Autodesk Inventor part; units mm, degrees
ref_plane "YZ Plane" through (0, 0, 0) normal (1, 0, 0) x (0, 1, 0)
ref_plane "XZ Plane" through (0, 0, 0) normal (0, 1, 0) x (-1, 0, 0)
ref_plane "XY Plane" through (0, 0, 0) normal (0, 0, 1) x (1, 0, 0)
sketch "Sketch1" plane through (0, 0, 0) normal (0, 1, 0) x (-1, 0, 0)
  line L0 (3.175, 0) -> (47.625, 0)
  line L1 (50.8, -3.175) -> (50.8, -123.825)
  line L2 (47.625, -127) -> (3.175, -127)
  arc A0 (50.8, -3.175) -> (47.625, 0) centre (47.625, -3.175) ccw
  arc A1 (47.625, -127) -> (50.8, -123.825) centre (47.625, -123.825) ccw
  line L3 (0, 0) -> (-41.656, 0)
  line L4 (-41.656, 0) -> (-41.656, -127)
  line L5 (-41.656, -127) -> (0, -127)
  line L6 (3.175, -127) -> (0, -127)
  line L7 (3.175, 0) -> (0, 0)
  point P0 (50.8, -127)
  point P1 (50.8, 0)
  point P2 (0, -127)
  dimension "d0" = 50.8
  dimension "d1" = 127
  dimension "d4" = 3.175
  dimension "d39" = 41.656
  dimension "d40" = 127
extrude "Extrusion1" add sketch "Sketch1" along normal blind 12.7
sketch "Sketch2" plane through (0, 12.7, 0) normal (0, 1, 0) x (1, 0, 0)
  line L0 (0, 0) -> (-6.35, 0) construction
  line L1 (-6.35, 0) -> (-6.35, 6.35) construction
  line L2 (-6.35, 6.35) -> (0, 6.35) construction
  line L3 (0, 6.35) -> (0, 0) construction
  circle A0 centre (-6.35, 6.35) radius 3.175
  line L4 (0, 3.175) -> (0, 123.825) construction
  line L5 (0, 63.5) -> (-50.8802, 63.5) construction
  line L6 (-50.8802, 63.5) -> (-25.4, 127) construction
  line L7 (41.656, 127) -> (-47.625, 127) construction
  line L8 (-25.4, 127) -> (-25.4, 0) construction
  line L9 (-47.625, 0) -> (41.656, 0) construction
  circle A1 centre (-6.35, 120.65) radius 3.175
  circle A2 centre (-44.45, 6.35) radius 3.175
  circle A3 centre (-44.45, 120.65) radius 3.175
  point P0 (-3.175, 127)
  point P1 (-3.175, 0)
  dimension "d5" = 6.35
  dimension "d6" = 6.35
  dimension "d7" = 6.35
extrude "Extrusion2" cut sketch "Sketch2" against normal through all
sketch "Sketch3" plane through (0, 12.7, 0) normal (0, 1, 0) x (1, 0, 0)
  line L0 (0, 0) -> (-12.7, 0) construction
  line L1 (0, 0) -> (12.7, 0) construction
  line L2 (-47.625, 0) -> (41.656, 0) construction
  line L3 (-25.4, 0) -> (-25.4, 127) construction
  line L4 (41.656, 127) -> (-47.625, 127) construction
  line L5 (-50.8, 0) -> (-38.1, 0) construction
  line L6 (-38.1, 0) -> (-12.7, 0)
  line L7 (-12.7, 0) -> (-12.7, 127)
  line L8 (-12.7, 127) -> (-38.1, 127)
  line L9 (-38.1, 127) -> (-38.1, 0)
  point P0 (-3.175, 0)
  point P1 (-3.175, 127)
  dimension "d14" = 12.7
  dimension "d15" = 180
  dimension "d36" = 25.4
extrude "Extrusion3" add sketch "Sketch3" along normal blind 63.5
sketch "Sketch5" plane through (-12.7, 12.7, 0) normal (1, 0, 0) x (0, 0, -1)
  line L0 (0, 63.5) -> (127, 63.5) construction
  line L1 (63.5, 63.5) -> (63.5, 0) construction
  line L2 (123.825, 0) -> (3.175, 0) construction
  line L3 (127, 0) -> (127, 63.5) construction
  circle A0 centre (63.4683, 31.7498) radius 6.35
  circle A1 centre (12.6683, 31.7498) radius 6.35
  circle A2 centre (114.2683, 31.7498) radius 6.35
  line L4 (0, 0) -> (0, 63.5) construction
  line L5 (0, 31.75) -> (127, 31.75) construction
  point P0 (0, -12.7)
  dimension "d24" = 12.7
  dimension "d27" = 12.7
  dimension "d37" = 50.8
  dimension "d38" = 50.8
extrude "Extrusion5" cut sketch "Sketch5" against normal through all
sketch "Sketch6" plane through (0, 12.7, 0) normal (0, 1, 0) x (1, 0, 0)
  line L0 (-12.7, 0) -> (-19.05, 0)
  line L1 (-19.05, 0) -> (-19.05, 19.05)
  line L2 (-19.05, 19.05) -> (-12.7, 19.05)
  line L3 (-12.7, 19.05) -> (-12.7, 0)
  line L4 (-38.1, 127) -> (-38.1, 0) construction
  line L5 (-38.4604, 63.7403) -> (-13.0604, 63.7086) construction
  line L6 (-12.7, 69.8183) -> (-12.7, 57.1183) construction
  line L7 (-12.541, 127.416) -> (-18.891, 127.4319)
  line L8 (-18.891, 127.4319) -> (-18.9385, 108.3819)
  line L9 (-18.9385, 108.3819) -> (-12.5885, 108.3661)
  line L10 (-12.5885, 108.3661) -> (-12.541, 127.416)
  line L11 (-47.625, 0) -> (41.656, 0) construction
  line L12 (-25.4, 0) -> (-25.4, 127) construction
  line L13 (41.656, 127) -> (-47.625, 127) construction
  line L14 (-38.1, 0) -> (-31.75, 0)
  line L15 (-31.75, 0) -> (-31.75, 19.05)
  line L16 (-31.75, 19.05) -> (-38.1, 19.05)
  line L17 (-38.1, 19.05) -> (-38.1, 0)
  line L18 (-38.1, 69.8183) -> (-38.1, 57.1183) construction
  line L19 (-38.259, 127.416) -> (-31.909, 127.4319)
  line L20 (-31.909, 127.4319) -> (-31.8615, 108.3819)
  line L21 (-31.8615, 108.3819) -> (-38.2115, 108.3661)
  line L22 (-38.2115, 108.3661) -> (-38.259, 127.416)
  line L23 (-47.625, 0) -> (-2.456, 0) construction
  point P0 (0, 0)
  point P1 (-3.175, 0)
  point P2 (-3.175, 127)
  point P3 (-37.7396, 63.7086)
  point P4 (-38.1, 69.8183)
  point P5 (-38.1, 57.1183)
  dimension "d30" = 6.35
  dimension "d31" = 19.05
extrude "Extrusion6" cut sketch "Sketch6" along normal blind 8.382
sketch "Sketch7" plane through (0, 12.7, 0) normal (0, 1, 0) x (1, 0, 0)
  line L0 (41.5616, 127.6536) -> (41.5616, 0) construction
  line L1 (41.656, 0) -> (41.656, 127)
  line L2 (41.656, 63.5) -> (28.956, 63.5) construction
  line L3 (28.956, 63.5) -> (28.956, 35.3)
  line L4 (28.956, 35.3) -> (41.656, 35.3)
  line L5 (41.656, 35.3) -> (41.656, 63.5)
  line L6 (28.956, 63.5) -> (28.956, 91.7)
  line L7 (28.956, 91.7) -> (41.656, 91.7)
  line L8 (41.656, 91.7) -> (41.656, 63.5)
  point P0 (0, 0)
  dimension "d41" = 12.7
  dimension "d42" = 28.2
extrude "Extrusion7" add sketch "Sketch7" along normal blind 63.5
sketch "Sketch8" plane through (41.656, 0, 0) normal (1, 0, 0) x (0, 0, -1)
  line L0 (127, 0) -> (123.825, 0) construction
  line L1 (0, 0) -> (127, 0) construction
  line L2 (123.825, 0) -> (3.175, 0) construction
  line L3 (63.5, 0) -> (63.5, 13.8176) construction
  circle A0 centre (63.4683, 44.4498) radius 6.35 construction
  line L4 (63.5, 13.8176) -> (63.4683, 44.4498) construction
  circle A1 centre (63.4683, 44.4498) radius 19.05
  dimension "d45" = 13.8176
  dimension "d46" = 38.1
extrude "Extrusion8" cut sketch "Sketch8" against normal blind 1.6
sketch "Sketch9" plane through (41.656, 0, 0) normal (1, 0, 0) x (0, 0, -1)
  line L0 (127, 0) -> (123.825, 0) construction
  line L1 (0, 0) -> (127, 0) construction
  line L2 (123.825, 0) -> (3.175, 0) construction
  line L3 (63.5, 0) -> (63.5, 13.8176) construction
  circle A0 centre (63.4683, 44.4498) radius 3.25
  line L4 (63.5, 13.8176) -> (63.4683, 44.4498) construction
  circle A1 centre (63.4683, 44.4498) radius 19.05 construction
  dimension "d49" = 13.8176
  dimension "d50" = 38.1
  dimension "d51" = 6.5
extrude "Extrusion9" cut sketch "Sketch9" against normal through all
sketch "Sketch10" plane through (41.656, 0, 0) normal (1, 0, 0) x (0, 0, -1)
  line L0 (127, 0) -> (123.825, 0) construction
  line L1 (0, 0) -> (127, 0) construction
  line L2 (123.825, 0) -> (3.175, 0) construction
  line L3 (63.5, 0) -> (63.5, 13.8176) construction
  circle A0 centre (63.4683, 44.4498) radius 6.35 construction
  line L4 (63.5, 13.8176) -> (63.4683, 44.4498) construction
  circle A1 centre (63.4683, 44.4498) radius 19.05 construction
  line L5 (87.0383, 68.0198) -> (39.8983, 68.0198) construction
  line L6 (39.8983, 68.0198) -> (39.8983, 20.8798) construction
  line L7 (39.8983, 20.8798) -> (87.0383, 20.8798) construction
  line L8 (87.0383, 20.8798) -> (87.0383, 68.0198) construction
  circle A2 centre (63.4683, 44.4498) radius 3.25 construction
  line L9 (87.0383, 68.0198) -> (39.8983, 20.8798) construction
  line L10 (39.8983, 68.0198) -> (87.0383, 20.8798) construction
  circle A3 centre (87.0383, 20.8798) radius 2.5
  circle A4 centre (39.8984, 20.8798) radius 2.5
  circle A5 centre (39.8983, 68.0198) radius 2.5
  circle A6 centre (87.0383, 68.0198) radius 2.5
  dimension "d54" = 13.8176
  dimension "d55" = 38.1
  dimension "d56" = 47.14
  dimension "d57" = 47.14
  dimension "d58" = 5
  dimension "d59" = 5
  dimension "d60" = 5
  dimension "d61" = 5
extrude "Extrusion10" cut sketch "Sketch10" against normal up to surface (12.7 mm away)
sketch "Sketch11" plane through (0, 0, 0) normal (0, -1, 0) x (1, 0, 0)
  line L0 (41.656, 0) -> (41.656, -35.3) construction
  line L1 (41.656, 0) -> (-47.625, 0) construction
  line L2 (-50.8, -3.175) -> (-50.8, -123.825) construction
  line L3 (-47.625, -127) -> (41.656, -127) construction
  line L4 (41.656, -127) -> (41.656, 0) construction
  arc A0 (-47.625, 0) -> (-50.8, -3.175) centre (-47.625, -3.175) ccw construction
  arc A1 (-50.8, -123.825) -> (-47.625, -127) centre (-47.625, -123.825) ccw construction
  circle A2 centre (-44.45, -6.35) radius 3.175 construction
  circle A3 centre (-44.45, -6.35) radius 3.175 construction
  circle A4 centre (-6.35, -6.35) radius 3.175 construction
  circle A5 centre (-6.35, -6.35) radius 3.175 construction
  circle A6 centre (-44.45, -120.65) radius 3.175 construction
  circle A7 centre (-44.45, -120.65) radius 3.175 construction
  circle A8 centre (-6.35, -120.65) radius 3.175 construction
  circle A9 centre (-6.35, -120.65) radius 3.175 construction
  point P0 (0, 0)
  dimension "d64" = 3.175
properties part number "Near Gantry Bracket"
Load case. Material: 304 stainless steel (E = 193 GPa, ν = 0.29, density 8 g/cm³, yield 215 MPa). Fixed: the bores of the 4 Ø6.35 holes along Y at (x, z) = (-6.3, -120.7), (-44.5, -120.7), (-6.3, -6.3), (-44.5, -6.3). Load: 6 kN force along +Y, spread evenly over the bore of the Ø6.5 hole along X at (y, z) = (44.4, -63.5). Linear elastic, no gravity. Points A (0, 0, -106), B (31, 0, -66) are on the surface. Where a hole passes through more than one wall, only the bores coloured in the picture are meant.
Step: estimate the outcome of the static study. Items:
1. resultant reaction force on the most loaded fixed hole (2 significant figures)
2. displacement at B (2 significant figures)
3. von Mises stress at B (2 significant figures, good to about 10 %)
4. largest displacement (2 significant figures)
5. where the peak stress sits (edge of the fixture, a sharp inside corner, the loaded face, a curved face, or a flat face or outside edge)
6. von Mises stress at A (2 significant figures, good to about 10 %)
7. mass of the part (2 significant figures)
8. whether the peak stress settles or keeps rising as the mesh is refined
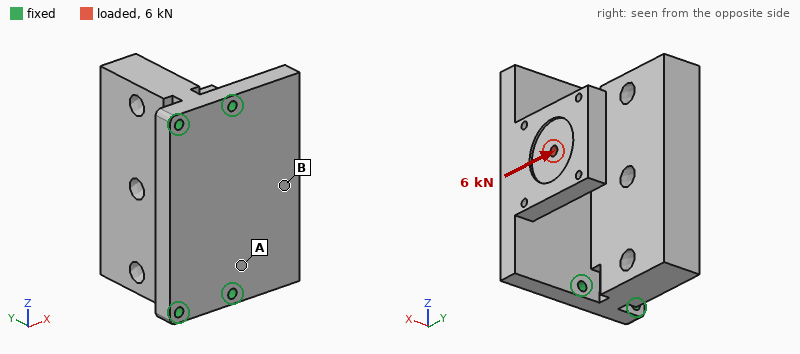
5.0 kN
0.068 mm
18 MPa
0.15 mm
edge of the fixture
61 MPa
3.0 kg
keeps rising
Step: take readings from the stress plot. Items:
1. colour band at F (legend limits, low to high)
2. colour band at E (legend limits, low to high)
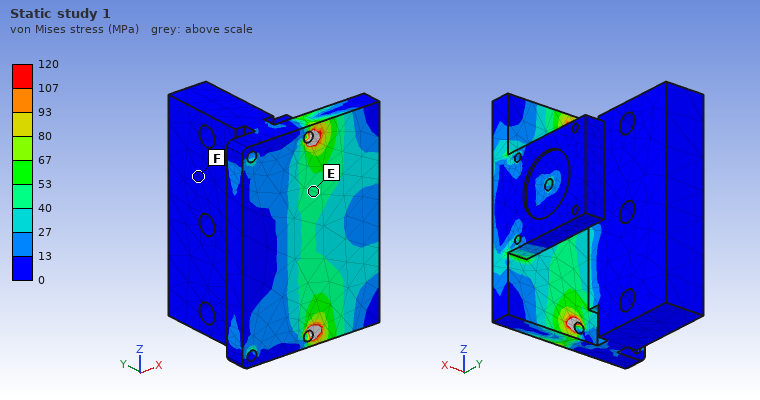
0 to 13 MPa
40 to 53 MPa
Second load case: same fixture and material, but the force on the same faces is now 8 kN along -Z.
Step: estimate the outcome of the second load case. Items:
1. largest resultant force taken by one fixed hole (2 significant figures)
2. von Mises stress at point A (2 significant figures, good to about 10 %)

5.2 kN
38 MPa
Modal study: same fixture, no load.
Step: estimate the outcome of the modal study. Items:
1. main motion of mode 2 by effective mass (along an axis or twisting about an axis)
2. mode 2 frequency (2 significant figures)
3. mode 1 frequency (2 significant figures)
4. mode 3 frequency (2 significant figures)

along X
2000 Hz
1200 Hz
2400 Hz
